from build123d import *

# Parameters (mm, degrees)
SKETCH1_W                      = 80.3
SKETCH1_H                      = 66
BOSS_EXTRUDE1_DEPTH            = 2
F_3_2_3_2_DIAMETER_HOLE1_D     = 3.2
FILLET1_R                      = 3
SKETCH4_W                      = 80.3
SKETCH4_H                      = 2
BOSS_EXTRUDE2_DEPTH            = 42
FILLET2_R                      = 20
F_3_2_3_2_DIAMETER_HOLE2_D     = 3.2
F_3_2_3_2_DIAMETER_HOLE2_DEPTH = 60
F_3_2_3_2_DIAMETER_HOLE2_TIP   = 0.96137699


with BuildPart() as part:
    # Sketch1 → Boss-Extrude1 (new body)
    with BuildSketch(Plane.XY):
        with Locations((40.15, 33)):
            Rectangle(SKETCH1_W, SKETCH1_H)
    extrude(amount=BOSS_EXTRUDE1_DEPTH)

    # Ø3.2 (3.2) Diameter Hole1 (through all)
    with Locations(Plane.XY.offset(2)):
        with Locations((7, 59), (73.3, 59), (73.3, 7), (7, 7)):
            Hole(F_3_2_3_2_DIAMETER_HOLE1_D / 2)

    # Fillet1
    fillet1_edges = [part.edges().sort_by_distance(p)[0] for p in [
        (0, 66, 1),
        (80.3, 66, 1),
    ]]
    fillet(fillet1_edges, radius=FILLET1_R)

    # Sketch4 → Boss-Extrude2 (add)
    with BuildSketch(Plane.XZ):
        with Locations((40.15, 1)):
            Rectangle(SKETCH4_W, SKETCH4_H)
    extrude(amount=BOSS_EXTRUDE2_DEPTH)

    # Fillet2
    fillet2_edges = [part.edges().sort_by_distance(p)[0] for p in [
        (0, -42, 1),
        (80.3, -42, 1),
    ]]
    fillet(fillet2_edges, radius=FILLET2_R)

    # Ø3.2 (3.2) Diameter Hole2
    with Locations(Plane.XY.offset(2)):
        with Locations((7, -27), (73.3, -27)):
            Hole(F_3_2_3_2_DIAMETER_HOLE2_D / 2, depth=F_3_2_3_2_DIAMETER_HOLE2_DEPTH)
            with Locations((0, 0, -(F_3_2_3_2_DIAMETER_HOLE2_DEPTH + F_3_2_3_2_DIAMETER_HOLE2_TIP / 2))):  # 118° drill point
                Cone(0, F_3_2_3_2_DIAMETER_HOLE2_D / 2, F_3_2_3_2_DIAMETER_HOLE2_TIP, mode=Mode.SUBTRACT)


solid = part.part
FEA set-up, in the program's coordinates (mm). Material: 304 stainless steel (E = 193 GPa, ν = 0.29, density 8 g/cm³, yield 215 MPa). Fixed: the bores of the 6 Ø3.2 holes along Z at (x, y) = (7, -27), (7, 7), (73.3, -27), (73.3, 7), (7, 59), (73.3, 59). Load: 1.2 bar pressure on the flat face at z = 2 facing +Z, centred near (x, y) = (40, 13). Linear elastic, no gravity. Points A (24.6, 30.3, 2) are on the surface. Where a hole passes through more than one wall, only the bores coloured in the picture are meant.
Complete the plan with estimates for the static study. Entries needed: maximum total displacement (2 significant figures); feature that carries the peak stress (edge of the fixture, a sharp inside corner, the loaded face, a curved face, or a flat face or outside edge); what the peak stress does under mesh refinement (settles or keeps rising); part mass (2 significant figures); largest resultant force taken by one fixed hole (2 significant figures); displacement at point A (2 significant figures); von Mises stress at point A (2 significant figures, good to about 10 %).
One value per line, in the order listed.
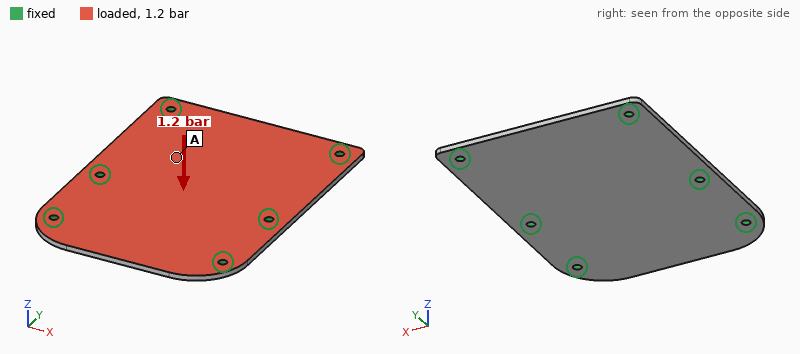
80 µm
edge of the fixture
keeps rising
140 g
210 N
63 µm
24 MPa
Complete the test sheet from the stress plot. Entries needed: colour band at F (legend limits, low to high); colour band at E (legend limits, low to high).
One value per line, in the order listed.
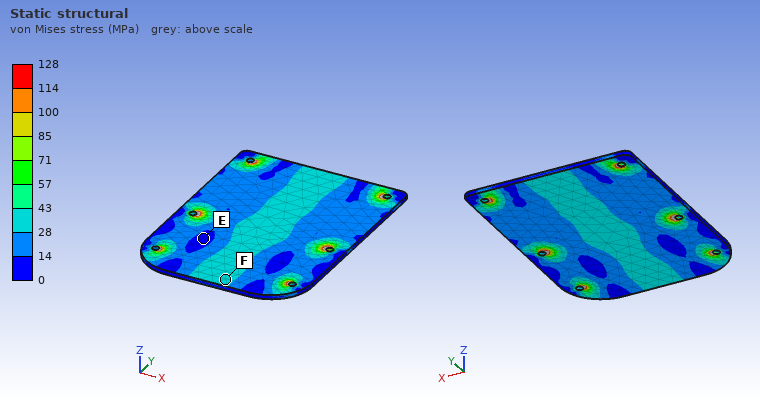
28 to 43 MPa
0 to 14 MPa
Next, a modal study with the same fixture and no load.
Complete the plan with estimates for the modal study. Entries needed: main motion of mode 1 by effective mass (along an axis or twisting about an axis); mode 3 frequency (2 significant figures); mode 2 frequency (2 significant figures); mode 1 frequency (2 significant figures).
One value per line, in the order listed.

along Z
2900 Hz
2200 Hz
1900 Hz
